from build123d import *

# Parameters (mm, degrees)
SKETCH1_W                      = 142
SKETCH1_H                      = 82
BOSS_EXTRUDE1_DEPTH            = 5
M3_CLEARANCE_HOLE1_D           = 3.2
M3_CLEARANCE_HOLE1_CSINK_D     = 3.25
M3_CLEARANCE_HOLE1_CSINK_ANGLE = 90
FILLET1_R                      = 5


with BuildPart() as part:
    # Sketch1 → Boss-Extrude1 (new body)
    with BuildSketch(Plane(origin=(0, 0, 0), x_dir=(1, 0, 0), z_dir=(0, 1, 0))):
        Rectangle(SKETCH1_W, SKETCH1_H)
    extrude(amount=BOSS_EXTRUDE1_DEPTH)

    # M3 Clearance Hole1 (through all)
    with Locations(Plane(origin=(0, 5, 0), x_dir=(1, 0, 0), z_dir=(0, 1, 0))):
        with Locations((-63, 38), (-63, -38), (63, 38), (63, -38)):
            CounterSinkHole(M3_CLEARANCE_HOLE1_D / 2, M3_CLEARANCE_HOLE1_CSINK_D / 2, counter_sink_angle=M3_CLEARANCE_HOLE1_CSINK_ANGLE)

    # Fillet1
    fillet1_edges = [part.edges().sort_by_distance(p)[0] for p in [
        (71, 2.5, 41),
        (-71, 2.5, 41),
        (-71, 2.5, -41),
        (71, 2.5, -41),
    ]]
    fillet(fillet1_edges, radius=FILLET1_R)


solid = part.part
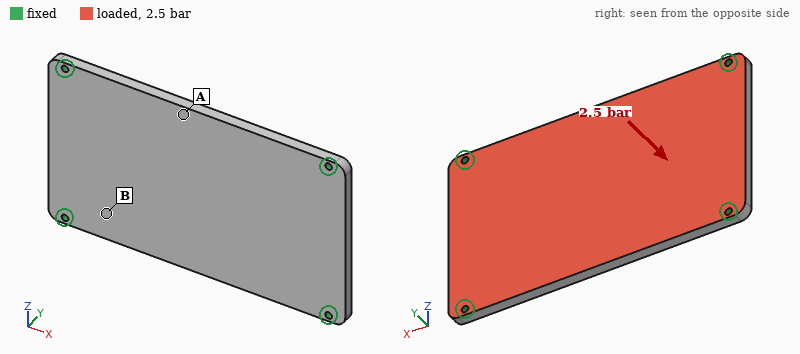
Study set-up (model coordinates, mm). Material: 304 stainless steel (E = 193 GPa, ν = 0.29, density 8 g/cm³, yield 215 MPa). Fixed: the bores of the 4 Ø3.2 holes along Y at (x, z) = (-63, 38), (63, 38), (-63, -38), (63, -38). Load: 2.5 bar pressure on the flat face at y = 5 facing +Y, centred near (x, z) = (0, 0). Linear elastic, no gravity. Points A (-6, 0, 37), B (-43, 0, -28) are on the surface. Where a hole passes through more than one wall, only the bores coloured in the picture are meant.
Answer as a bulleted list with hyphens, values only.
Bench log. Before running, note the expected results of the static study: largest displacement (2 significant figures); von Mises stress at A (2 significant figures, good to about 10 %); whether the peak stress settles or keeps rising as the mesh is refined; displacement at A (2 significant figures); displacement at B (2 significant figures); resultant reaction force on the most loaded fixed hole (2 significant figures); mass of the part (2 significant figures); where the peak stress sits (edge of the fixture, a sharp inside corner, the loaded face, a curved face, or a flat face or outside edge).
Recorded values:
- 0.15 mm
- 57 MPa
- keeps rising
- 0.14 mm
- 0.058 mm
- 720 N
- 460 g
- edge of the fixture
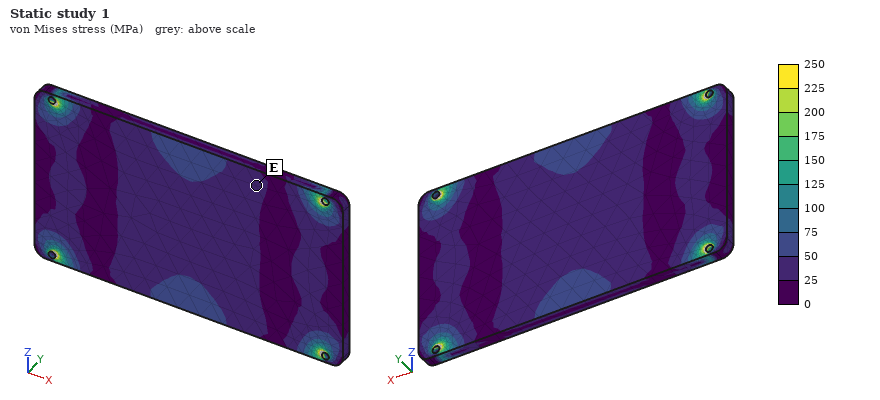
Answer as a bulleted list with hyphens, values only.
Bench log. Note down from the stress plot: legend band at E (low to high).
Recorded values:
- 25 to 50 MPa
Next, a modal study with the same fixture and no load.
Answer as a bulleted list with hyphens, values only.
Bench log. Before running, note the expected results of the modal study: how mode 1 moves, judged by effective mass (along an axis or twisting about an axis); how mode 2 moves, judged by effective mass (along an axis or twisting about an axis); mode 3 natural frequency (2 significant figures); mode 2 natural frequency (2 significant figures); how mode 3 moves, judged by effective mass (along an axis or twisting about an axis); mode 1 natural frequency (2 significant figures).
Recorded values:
- along Y
- twisting about X
- 3100 Hz
- 2100 Hz
- twisting about Z
- 1200 Hz
